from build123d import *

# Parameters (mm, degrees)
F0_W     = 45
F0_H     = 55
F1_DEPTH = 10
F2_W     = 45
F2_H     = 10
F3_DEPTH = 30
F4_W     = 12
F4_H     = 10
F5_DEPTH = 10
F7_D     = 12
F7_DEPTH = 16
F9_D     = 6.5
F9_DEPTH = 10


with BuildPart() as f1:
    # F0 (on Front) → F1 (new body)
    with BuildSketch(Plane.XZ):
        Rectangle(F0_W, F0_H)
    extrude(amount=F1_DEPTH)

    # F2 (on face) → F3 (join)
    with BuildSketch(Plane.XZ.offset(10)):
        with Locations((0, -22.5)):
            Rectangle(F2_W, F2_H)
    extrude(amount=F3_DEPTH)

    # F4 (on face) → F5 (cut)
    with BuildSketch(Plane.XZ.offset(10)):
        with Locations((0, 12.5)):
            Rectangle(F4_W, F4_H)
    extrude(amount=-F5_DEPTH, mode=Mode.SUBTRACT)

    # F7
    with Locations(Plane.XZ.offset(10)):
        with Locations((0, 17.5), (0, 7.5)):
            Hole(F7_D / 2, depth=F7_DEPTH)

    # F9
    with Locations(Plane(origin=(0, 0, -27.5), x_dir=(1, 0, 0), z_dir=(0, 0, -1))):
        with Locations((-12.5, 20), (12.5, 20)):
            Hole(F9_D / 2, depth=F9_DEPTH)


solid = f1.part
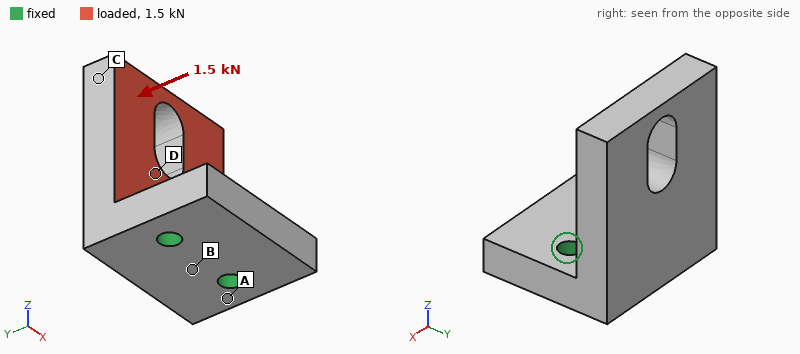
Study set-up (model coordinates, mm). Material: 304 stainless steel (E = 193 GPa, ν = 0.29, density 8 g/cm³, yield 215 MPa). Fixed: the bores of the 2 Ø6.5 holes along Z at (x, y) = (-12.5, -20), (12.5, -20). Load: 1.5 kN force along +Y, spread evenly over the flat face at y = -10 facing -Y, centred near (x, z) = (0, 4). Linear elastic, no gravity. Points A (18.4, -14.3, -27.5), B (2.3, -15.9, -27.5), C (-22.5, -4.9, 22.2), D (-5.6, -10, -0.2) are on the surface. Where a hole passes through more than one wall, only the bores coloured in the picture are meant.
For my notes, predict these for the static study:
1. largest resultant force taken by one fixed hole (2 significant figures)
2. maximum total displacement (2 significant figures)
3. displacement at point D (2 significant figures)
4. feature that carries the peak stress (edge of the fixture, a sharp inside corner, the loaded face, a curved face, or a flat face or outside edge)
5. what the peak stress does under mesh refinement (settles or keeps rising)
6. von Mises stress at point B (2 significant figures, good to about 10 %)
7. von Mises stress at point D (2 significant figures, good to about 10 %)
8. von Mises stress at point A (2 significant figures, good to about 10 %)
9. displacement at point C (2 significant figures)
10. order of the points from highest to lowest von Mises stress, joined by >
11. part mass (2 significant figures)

770 N
67 µm
24 µm
edge of the fixture
keeps rising
31 MPa
19 MPa
43 MPa
57 µm
A > B > D > C
280 g
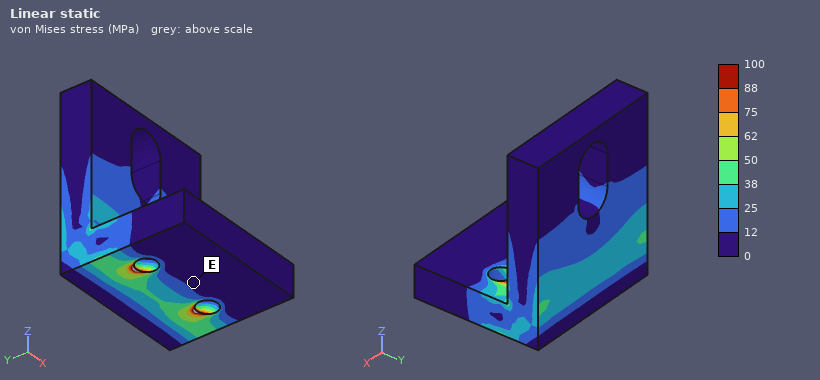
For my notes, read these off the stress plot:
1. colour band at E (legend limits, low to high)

0 to 12 MPa
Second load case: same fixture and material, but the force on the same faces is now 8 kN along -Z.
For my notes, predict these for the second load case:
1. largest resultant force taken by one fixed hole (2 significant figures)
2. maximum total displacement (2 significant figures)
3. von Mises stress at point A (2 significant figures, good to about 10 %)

4.0 kN
25 µm
33 MPa
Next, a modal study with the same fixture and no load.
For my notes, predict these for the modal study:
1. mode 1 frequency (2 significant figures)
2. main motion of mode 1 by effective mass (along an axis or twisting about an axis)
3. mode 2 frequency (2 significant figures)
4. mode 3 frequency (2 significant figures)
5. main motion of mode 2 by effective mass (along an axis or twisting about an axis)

2400 Hz
along Y
4900 Hz
6700 Hz
along X
